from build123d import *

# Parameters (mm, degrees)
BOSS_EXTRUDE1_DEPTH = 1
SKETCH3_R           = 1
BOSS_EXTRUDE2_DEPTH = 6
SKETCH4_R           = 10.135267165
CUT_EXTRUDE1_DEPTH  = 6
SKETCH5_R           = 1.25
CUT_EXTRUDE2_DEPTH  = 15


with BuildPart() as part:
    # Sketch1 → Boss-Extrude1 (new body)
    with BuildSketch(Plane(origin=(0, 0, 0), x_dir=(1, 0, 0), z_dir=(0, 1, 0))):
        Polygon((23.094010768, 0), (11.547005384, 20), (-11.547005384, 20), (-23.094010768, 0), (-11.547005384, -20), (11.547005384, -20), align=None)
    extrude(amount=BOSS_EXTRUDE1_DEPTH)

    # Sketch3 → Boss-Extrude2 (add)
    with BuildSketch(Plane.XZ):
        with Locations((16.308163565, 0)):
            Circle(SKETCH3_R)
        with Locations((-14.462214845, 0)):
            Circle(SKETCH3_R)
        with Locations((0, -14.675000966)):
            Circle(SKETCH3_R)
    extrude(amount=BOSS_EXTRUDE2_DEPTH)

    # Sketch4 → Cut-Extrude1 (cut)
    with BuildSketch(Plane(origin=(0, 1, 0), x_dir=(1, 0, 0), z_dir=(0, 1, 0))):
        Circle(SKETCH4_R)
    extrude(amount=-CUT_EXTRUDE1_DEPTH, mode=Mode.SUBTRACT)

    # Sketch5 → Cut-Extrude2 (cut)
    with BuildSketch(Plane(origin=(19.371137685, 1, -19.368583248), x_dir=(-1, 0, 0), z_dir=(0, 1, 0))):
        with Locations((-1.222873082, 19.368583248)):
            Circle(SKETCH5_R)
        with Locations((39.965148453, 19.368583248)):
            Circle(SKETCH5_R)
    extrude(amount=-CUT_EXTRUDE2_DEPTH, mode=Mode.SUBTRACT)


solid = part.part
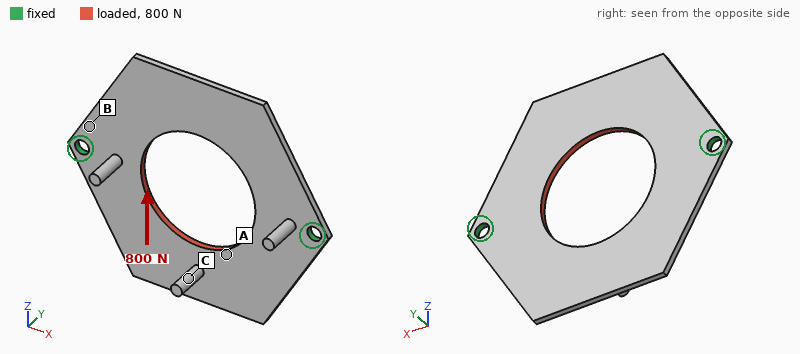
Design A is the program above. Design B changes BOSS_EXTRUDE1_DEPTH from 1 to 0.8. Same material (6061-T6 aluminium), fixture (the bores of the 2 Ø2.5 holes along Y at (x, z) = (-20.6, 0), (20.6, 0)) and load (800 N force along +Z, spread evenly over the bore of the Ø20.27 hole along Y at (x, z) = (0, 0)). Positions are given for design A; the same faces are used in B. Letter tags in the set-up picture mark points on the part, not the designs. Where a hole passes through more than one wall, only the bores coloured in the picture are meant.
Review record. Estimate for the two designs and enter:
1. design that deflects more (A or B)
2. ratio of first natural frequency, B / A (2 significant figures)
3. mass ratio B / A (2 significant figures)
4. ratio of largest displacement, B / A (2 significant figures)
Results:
B
0.81
0.81
1.3
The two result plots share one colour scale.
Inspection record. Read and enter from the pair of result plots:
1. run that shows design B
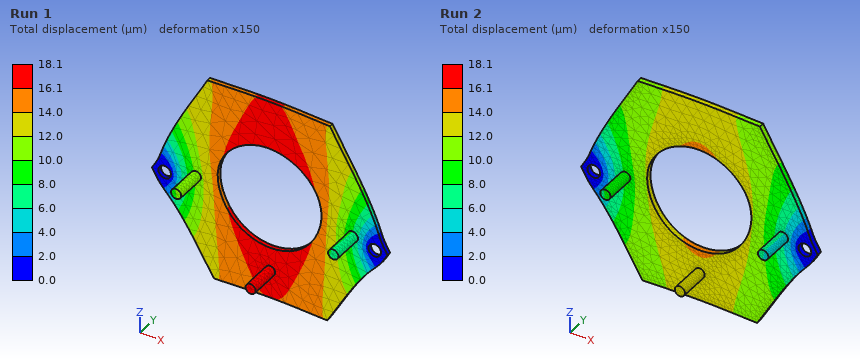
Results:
Run 1
